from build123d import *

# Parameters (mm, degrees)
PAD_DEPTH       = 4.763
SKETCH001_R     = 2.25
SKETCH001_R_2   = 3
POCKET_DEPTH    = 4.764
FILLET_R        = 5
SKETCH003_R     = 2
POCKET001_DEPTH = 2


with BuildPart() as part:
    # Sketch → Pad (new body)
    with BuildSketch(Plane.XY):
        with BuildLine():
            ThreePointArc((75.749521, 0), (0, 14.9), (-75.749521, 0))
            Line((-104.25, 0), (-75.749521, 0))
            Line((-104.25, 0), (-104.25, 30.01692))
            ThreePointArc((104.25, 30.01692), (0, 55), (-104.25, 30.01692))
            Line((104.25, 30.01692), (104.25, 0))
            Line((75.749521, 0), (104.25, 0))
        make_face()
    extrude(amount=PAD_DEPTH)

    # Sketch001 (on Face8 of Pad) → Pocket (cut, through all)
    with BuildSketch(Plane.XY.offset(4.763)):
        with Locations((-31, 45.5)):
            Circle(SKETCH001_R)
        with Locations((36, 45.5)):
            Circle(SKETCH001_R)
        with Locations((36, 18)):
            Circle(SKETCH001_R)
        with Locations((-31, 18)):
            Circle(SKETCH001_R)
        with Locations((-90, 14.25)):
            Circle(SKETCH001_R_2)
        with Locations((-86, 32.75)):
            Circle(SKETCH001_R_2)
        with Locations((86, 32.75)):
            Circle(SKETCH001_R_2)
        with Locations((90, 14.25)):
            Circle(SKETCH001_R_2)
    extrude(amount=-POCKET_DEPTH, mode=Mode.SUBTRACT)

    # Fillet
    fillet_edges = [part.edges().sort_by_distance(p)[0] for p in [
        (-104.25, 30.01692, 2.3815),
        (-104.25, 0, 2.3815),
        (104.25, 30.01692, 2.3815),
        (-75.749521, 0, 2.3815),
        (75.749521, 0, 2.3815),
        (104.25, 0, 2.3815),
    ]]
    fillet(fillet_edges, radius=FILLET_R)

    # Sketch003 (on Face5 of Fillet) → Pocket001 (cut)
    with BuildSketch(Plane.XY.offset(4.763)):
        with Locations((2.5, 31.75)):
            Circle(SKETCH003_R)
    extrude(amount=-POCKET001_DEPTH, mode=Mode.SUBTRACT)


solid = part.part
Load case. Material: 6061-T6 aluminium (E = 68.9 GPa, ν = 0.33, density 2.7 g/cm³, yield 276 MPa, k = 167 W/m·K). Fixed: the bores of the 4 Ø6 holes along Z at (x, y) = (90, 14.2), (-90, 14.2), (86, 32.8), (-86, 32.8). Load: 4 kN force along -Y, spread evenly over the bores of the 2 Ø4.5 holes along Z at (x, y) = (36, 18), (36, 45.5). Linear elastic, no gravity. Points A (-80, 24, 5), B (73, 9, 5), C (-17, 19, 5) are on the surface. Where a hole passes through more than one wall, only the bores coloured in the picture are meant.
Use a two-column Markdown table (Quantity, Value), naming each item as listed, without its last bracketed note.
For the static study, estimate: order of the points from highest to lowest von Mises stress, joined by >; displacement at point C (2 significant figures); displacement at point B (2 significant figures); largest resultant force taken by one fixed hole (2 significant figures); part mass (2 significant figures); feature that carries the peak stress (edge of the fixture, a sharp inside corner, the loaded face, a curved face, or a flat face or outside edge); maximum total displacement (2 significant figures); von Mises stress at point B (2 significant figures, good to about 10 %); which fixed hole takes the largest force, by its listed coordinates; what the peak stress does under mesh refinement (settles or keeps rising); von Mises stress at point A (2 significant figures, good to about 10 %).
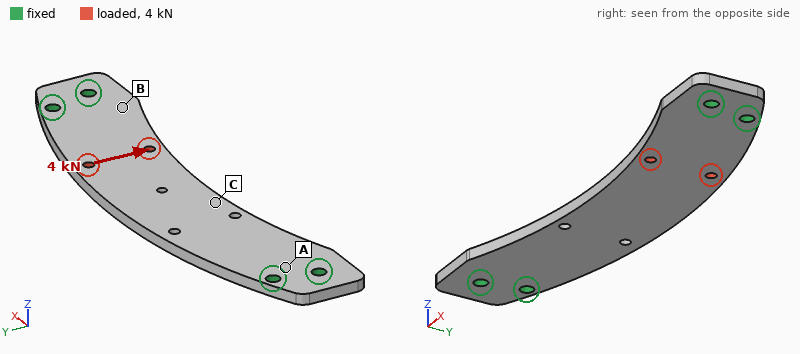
| Quantity | Value |
|---|---|
| order of the points from highest to lowest von Mises stress, joined by > | B > A > C |
| displacement at point C | 56 µm |
| displacement at point B | 24 µm |
| largest resultant force taken by one fixed hole | 4.3 kN |
| part mass | 100 g |
| feature that carries the peak stress | edge of the fixture |
| maximum total displacement | 80 µm |
| von Mises stress at point B | 31 MPa |
| which fixed hole takes the largest force, by its listed coordinates | (90, 14.2) |
| what the peak stress does under mesh refinement | keeps rising |
| von Mises stress at point A | 18 MPa |
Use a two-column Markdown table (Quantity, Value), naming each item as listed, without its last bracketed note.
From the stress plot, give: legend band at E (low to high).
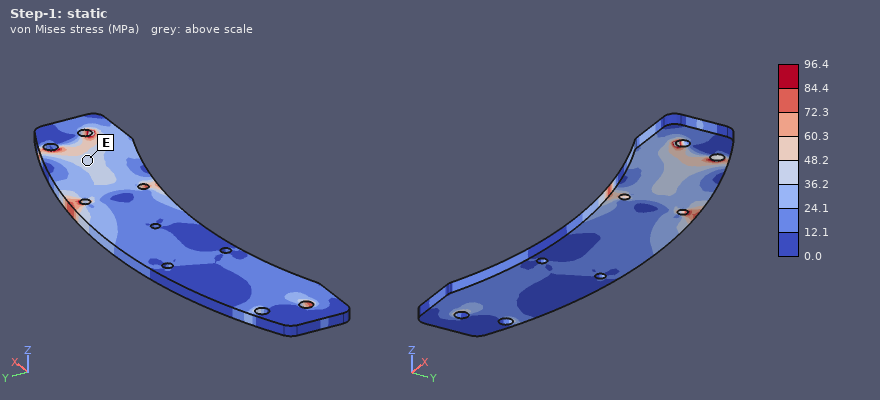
| Quantity | Value |
|---|---|
| legend band at E | 36.2 to 48.2 MPa |
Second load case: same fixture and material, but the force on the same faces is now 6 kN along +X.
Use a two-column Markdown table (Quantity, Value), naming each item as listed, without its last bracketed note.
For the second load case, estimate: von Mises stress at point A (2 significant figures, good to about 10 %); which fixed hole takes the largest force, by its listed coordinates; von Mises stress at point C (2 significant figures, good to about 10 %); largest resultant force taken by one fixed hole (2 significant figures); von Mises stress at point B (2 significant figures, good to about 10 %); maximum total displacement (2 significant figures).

| Quantity | Value |
|---|---|
| von Mises stress at point A | 7.8 MPa |
| which fixed hole takes the largest force, by its listed coordinates | (86, 32.8) |
| von Mises stress at point C | 11 MPa |
| largest resultant force taken by one fixed hole | 2.5 kN |
| von Mises stress at point B | 13 MPa |
| maximum total displacement | 23 µm |
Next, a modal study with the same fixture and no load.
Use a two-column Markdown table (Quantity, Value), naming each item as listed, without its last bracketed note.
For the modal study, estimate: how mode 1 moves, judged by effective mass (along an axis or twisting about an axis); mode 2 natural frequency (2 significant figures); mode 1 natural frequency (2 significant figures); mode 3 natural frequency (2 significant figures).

| Quantity | Value |
|---|---|
| how mode 1 moves, judged by effective mass | along Z |
| mode 2 natural frequency | 2200 Hz |
| mode 1 natural frequency | 820 Hz |
| mode 3 natural frequency | 2200 Hz |
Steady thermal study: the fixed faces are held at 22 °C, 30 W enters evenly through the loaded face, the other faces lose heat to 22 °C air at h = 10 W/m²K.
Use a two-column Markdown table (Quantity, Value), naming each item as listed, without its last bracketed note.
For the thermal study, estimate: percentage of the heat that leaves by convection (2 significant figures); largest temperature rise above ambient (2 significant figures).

| Quantity | Value |
|---|---|
| percentage of the heat that leaves by convection | 8.5 % |
| largest temperature rise above ambient | 36 K |
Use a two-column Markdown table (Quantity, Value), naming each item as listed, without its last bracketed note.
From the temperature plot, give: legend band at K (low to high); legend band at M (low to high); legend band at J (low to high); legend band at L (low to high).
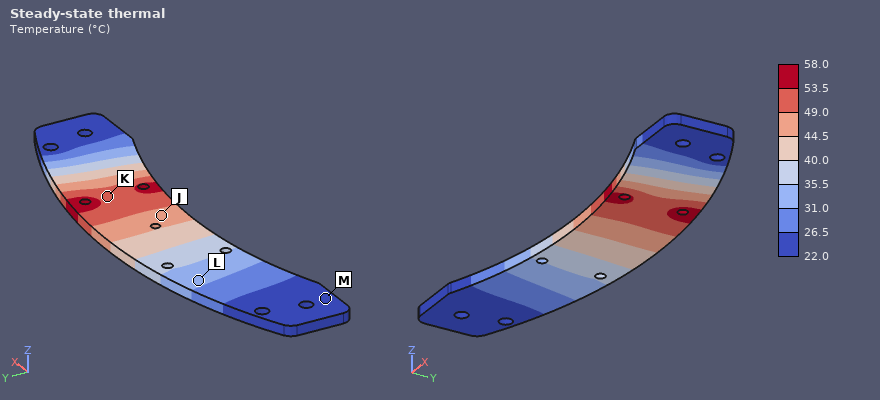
| Quantity | Value |
|---|---|
| legend band at K | 49.0 to 53.5 °C |
| legend band at M | 22.0 to 26.5 °C |
| legend band at J | 44.5 to 49.0 °C |
| legend band at L | 31.0 to 35.5 °C |
